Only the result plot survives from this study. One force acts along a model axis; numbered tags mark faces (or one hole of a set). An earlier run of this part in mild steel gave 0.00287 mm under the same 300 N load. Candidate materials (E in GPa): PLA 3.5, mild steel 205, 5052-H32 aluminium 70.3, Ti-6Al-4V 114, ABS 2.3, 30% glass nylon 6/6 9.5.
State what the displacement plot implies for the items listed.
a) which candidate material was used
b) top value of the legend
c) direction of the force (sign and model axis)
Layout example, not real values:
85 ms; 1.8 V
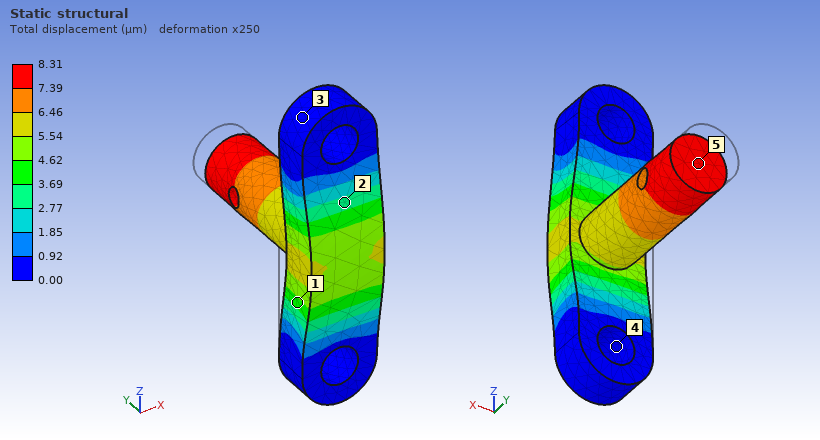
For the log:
5052-H32 aluminium; 8.31 µm; -Y
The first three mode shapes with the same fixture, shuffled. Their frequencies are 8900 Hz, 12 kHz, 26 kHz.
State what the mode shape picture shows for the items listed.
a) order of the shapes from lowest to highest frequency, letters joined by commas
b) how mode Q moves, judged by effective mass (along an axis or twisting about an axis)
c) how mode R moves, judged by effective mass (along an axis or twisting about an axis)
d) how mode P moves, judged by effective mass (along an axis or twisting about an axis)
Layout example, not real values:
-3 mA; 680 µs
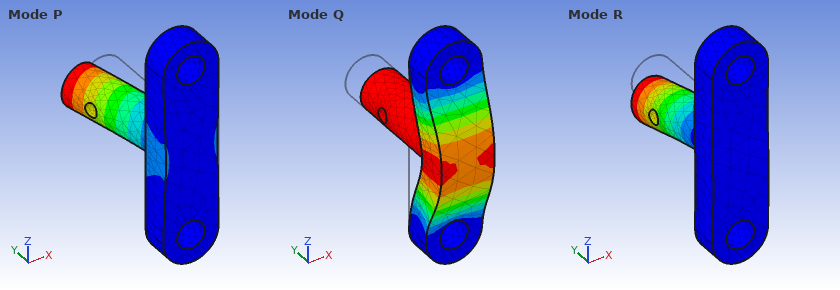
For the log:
P, R, Q; along Y; along Z; along X
